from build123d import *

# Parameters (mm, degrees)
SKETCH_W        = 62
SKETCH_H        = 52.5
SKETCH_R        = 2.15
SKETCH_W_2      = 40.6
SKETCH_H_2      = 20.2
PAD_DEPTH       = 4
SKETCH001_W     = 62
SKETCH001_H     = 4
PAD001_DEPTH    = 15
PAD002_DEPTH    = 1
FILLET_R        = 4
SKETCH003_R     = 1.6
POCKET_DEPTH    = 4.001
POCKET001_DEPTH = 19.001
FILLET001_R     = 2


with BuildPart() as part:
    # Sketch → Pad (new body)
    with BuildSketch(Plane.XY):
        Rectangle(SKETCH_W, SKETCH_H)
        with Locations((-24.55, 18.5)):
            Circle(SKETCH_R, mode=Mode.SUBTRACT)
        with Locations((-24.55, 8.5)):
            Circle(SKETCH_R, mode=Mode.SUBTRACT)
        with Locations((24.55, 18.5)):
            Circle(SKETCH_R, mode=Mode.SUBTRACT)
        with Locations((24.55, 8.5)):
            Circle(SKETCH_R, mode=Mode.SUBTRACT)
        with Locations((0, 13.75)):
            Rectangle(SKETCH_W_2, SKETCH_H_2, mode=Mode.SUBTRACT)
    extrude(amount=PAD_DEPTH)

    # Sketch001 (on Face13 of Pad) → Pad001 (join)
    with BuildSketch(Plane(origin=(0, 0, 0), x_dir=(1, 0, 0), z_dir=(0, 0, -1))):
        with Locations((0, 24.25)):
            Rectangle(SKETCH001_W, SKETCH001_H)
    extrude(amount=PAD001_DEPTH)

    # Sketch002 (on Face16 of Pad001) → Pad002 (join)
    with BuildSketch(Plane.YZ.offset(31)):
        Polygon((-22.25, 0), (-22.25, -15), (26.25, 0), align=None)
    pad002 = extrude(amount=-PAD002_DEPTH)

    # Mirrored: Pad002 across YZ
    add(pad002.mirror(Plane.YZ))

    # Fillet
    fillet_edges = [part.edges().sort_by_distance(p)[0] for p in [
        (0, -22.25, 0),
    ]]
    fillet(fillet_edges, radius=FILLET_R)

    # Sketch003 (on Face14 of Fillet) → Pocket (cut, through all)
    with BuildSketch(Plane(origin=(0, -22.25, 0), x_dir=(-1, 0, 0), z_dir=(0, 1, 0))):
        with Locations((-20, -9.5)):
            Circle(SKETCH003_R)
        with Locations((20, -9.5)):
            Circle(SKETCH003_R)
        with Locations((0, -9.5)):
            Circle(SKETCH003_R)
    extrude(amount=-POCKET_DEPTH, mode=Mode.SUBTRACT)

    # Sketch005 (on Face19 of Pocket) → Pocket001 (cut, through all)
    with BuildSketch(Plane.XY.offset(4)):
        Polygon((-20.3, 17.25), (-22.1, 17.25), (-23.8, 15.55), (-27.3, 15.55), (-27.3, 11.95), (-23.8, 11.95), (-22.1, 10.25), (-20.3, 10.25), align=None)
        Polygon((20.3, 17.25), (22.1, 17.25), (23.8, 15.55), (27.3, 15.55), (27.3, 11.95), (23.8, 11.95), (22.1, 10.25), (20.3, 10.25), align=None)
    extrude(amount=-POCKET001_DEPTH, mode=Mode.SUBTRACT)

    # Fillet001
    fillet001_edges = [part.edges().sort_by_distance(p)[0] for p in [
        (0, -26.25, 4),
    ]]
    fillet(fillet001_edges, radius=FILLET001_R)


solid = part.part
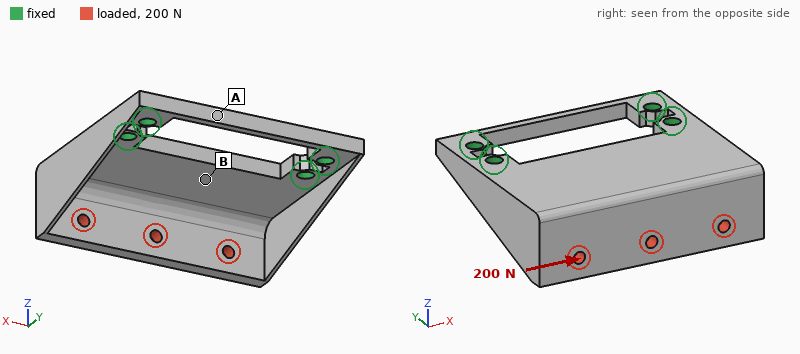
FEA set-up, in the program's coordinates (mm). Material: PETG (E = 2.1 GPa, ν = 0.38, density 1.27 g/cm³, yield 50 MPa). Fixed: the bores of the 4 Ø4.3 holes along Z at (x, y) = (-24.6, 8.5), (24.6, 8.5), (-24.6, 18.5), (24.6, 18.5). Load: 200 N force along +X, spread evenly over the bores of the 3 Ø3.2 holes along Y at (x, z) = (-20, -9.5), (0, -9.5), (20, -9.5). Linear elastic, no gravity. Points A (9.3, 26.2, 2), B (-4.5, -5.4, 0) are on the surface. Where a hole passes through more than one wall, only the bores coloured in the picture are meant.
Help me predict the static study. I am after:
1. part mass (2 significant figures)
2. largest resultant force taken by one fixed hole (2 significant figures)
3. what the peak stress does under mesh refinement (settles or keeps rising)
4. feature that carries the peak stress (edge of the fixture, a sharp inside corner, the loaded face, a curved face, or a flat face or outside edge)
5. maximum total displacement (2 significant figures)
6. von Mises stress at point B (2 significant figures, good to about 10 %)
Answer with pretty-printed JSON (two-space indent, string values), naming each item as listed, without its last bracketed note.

{
  "part mass": "17 g",
  "largest resultant force taken by one fixed hole": "170 N",
  "what the peak stress does under mesh refinement": "keeps rising",
  "feature that carries the peak stress": "edge of the fixture",
  "maximum total displacement": "0.89 mm",
  "von Mises stress at point B": "6.0 MPa"
}
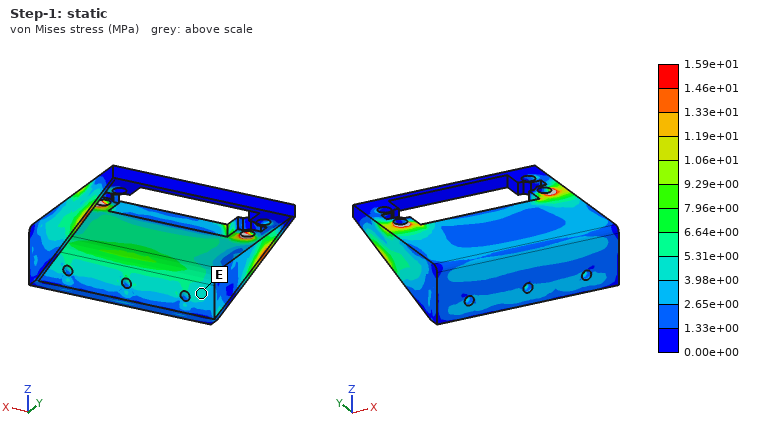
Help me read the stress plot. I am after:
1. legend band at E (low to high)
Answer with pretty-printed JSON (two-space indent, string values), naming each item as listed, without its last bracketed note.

{
  "legend band at E": "3.98e+00 to 5.31e+00 MPa"
}
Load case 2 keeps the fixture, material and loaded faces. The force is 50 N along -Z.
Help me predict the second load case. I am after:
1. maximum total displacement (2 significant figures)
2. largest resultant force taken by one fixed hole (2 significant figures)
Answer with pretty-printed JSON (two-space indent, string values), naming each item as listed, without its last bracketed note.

{
  "maximum total displacement": "0.90 mm",
  "largest resultant force taken by one fixed hole": "58 N"
}
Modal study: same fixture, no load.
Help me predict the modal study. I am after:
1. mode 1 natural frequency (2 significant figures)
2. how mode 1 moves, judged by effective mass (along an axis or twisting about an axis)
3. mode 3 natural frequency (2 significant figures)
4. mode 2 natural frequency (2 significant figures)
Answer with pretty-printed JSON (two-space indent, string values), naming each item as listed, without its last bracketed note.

{
  "mode 1 natural frequency": "440 Hz",
  "how mode 1 moves, judged by effective mass": "along Z",
  "mode 3 natural frequency": "1700 Hz",
  "mode 2 natural frequency": "850 Hz"
}
